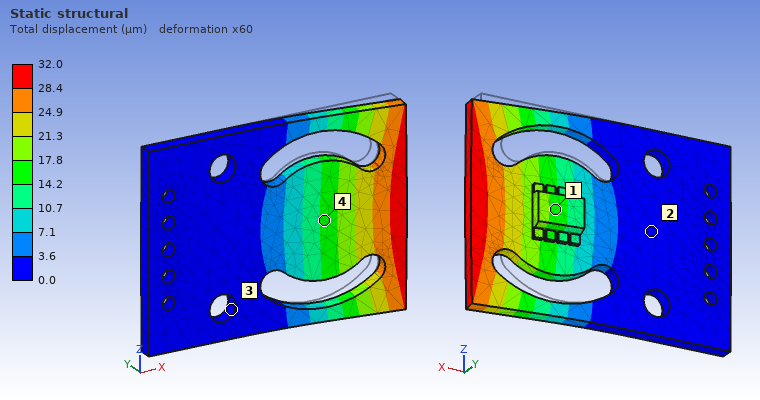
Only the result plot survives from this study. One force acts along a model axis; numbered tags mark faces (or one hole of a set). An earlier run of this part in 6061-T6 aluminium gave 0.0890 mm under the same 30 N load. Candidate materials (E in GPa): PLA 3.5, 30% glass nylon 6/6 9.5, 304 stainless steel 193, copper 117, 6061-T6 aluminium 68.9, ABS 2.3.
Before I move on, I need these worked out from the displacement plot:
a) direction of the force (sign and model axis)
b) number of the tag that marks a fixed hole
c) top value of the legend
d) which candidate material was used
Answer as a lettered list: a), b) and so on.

a) -Y
b) 3
c) 32.0 µm
d) 304 stainless steel
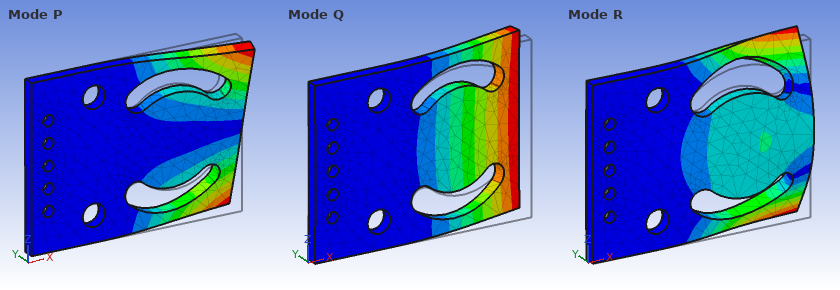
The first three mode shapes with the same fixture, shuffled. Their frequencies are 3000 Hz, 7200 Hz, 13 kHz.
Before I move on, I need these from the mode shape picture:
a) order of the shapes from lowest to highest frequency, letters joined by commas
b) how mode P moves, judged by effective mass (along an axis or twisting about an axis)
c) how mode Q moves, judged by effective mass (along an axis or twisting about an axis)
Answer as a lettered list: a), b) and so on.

a) Q, P, R
b) twisting about X
c) along Y
